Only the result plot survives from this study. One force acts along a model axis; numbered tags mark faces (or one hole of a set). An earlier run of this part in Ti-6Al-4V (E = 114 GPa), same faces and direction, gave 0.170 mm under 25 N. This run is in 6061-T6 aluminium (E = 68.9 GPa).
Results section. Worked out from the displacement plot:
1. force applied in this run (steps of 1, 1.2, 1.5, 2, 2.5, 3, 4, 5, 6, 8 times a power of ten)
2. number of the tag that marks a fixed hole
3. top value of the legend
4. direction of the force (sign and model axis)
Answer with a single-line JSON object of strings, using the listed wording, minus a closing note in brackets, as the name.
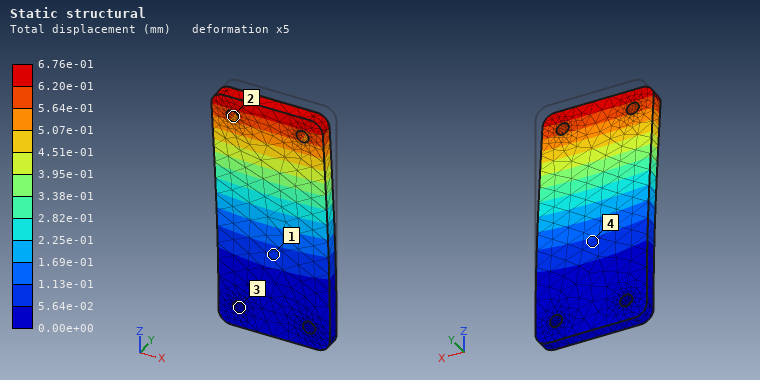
{"force applied in this run": "60 N", "number of the tag that marks a fixed hole": "3", "top value of the legend": "6.76e-01 mm", "direction of the force": "-Y"}
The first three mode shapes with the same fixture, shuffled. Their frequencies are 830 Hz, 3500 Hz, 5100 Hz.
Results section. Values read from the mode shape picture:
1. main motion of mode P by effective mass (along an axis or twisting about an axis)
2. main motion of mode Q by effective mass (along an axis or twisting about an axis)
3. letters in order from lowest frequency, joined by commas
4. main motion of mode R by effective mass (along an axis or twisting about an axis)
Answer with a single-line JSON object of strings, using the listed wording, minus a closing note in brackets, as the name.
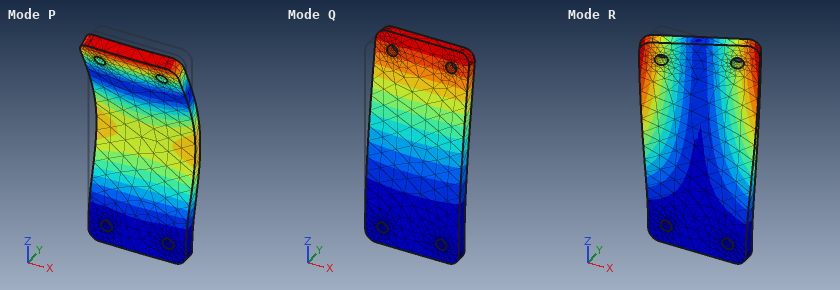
{"main motion of mode P by effective mass": "along Y", "main motion of mode Q by effective mass": "along Y", "letters in order from lowest frequency, joined by commas": "Q, R, P", "main motion of mode R by effective mass": "twisting about Z"}
